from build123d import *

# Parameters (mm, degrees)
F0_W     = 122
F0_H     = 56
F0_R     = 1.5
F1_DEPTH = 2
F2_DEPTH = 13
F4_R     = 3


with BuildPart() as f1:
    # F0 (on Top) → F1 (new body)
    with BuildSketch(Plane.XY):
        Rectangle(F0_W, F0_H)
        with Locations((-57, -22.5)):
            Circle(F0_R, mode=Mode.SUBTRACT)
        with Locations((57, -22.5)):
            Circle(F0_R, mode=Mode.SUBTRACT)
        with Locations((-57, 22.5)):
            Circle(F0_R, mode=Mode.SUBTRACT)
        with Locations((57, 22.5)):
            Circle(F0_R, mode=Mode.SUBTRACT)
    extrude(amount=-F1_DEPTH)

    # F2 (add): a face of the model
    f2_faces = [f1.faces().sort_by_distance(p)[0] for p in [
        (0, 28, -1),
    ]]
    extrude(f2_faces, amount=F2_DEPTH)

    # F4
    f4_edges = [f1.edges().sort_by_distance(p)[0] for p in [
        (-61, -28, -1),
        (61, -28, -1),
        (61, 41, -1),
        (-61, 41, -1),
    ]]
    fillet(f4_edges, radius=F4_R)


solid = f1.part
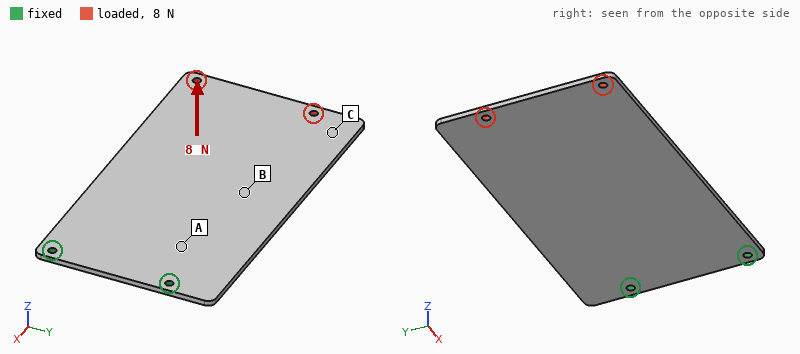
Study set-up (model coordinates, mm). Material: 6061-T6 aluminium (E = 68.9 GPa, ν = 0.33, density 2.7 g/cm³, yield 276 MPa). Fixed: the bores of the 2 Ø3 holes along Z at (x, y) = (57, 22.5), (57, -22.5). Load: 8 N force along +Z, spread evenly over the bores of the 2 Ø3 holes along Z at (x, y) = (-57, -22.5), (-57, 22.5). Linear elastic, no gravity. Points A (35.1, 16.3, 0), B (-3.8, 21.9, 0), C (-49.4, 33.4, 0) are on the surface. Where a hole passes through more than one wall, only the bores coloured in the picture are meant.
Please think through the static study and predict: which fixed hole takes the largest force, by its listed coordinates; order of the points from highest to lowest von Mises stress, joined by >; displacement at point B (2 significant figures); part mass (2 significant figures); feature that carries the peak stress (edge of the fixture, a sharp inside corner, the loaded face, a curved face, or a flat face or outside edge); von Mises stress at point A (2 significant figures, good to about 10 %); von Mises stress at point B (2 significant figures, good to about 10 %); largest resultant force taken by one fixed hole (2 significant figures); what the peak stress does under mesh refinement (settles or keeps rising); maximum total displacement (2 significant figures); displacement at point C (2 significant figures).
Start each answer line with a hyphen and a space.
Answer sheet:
- (57, 22.5)
- A > B > C
- 0.51 mm
- 45 g
- edge of the fixture
- 14 MPa
- 9.1 MPa
- 5.1 N
- keeps rising
- 1.5 mm
- 1.2 mm
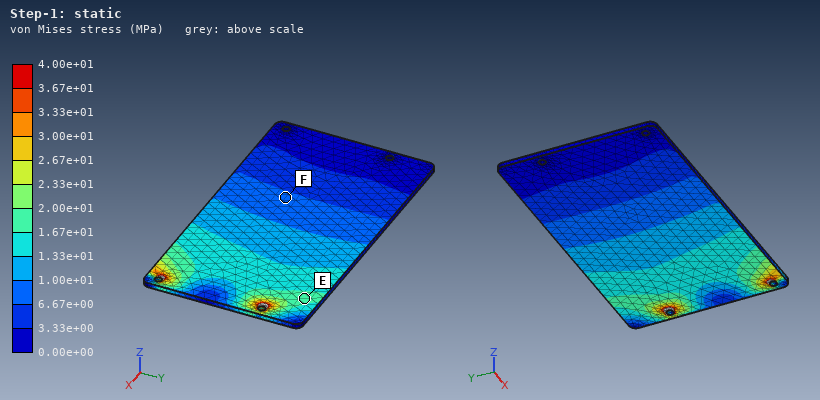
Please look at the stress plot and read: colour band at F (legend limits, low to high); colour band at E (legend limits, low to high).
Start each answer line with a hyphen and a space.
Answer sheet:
- 6.67e+00 to 1.00e+01 MPa
- 1.67e+01 to 2.00e+01 MPa
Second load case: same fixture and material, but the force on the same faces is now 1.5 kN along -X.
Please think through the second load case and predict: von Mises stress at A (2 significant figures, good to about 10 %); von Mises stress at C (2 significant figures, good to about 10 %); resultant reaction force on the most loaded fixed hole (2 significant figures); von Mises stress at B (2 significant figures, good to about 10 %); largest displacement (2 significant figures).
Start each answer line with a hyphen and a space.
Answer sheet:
- 12 MPa
- 7.6 MPa
- 770 N
- 8.0 MPa
- 42 µm
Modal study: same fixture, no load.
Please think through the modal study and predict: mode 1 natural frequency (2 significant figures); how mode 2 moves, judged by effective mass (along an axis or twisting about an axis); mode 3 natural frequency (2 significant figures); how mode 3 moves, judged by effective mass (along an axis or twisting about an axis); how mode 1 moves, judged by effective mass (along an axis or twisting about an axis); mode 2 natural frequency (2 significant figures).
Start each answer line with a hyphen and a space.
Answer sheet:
- 110 Hz
- twisting about X
- 700 Hz
- along Z
- along Z
- 430 Hz
